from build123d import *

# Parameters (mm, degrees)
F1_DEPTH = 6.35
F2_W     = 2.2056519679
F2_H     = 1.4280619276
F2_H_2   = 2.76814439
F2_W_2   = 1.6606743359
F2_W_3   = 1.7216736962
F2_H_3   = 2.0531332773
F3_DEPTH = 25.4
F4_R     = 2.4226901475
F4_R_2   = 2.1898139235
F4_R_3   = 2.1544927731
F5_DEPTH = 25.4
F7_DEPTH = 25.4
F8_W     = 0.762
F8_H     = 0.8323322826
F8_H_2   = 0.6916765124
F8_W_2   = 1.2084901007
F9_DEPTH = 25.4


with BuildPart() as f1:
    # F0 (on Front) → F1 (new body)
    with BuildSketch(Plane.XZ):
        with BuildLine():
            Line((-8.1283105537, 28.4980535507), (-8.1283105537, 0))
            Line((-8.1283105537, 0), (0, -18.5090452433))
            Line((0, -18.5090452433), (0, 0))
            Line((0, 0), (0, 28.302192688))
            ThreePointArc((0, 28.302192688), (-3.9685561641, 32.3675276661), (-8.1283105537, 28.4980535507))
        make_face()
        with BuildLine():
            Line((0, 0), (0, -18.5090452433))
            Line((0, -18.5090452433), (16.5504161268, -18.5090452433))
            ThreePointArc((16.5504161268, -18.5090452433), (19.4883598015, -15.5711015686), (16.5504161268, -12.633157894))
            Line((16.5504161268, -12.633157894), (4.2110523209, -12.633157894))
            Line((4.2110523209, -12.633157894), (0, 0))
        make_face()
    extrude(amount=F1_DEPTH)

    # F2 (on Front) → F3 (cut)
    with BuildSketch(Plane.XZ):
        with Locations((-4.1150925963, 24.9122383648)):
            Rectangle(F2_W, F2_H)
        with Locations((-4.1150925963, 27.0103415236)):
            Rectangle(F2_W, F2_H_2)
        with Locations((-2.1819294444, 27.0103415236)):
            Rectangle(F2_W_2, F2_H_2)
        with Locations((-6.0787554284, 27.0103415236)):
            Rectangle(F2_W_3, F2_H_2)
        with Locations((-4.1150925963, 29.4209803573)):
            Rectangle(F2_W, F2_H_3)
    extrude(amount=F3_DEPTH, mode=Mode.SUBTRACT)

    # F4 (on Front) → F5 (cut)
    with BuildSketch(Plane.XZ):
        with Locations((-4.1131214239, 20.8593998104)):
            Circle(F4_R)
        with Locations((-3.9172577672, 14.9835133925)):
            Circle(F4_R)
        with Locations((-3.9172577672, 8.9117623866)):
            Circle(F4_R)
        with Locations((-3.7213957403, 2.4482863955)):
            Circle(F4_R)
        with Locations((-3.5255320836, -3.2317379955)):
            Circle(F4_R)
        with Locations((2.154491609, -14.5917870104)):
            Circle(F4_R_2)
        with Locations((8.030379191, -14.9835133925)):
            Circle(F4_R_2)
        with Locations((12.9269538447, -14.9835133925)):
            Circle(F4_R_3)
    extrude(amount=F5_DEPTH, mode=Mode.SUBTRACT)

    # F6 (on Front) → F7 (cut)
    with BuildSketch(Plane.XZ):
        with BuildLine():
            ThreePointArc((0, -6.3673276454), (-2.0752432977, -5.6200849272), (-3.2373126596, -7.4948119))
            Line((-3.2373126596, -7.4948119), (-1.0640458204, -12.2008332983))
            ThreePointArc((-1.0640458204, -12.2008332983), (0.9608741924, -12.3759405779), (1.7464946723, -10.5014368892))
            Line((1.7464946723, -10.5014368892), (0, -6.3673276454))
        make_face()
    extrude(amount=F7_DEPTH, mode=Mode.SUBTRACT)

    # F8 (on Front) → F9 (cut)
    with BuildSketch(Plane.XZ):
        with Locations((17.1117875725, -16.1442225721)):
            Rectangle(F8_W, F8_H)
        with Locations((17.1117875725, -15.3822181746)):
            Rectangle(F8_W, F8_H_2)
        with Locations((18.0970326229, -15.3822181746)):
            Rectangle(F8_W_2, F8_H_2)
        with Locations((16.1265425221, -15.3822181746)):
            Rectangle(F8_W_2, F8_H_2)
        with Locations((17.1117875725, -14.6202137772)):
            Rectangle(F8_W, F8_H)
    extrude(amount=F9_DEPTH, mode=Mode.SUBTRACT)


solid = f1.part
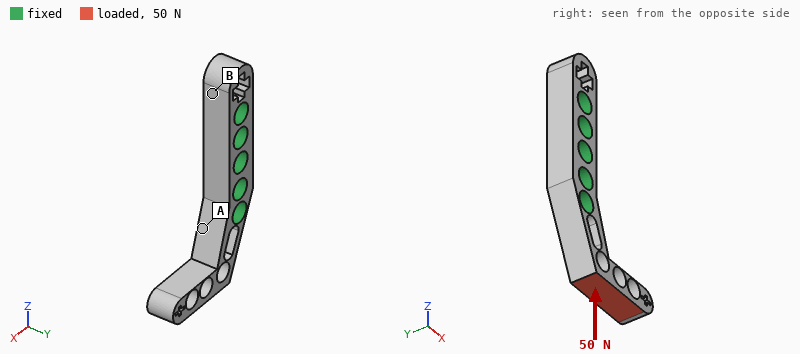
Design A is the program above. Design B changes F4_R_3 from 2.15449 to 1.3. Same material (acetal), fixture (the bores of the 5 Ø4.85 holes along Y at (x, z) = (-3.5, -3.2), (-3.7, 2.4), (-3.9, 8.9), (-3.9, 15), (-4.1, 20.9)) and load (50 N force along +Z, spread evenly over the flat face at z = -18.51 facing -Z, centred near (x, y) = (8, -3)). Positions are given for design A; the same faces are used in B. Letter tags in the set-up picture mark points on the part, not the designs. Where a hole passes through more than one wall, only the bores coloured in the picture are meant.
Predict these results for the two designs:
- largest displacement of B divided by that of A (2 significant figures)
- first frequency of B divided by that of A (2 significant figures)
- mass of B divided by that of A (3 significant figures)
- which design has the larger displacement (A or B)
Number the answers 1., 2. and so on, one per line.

1. 0.90
2. 0.92
3. 1.03
4. A
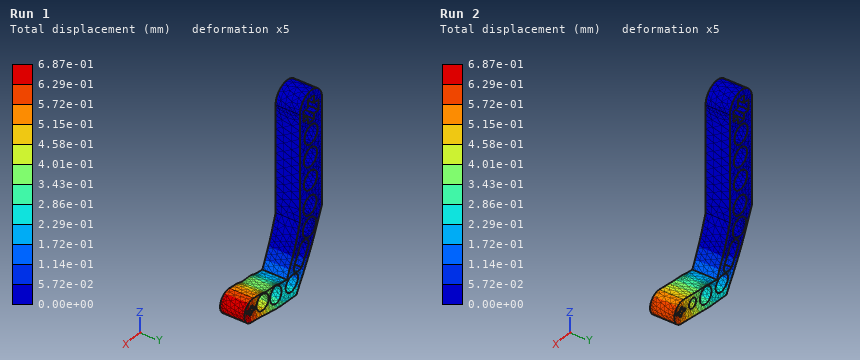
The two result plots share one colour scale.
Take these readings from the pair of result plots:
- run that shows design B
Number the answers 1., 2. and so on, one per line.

1. Run 2
